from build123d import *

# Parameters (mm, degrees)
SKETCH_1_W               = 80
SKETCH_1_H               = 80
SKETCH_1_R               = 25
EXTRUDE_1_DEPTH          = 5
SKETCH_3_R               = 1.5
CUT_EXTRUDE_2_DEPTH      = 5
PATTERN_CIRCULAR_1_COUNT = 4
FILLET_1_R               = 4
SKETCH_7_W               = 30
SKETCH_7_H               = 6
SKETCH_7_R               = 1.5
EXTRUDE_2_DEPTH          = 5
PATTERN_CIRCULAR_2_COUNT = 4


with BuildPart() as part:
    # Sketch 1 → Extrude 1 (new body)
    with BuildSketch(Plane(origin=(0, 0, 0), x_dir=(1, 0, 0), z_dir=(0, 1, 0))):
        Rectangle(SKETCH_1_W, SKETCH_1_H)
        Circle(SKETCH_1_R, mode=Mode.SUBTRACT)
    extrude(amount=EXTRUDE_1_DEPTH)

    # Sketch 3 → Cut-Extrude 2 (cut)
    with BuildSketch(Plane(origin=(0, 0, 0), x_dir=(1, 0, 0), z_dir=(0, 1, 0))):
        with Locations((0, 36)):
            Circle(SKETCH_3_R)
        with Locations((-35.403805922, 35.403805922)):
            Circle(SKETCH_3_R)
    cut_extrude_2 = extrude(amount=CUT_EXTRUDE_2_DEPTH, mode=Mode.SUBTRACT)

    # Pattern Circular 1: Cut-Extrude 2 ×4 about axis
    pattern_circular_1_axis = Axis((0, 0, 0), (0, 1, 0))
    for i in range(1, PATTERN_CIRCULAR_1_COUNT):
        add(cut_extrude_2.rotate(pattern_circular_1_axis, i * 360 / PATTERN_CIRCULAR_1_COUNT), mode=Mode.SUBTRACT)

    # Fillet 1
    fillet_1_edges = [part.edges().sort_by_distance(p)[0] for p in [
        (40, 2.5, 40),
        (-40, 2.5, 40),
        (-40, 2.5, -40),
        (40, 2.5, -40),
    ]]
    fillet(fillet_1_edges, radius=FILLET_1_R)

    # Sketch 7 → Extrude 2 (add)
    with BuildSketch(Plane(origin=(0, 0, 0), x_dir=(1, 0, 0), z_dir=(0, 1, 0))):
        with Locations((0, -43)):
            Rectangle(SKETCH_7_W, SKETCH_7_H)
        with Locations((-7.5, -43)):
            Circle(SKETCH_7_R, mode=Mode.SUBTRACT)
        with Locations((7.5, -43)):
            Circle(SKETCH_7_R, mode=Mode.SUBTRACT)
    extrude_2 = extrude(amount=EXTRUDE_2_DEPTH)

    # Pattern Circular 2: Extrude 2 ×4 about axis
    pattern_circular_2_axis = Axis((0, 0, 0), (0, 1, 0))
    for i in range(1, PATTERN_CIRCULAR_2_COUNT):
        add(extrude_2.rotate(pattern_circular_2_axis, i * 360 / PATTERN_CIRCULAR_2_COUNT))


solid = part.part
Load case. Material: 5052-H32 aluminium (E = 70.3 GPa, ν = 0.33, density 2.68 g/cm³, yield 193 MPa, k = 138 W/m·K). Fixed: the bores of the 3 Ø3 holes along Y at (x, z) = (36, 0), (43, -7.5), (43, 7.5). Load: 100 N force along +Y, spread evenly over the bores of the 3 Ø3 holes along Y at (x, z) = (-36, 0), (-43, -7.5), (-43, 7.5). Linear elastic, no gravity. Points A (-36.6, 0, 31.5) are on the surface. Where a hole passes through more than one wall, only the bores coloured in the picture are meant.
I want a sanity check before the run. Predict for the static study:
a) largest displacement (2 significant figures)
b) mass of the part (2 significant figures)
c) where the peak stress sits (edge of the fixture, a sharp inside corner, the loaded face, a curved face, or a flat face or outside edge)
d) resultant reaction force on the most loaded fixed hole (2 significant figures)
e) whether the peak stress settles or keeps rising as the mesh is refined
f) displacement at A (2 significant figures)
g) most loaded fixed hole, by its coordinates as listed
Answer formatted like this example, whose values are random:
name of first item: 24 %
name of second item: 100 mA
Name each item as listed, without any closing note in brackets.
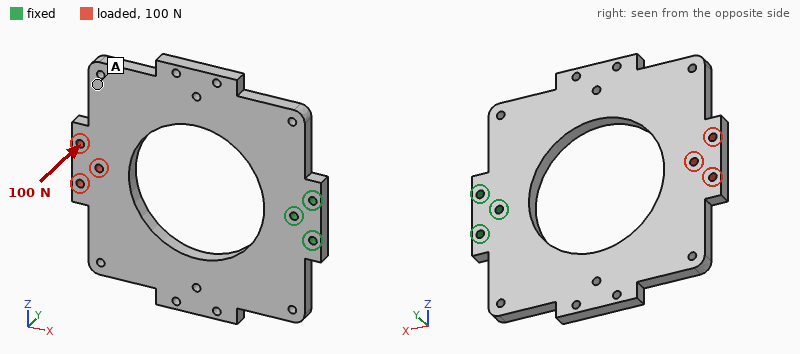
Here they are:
largest displacement: 0.77 mm
mass of the part: 67 g
where the peak stress sits: edge of the fixture
resultant reaction force on the most loaded fixed hole: 510 N
whether the peak stress settles or keeps rising as the mesh is refined: keeps rising
displacement at A: 0.64 mm
most loaded fixed hole, by its coordinates as listed: (36, 0)
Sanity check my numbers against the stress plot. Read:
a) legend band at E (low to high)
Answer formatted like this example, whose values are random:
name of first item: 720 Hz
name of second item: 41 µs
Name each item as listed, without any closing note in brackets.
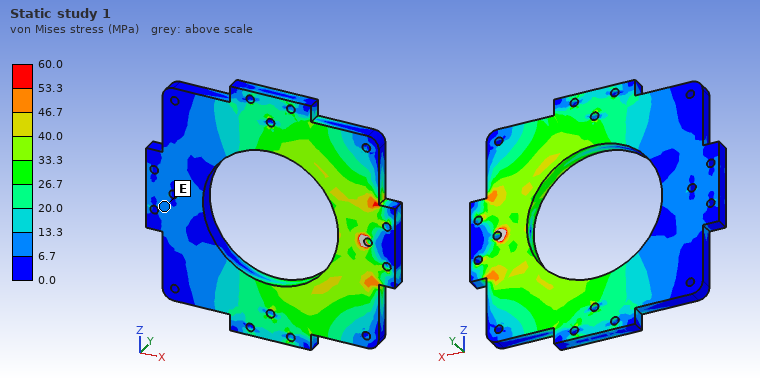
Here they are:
legend band at E: 6.7 to 13.3 MPa
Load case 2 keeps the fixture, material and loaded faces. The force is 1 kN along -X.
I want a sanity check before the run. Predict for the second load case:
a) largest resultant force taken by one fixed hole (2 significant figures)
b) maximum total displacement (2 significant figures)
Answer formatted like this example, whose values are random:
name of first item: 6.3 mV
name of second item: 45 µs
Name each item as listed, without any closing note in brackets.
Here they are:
largest resultant force taken by one fixed hole: 670 N
maximum total displacement: 35 µm
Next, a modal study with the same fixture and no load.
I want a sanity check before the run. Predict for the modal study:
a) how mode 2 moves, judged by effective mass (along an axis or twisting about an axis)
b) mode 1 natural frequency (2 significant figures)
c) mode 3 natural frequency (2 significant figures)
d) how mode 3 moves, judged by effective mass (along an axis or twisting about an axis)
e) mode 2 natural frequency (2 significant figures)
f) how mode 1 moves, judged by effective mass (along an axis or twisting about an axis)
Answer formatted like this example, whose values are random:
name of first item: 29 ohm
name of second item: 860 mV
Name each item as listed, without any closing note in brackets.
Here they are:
how mode 2 moves, judged by effective mass: twisting about X
mode 1 natural frequency: 430 Hz
mode 3 natural frequency: 1700 Hz
how mode 3 moves, judged by effective mass: along Z
mode 2 natural frequency: 820 Hz
how mode 1 moves, judged by effective mass: along Y
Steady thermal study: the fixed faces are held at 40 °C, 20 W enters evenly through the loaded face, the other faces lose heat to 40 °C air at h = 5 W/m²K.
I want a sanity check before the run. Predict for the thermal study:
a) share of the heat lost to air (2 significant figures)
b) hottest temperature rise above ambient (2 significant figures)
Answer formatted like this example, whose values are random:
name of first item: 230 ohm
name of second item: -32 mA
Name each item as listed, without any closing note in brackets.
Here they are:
share of the heat lost to air: 11 %
hottest temperature rise above ambient: 72 K
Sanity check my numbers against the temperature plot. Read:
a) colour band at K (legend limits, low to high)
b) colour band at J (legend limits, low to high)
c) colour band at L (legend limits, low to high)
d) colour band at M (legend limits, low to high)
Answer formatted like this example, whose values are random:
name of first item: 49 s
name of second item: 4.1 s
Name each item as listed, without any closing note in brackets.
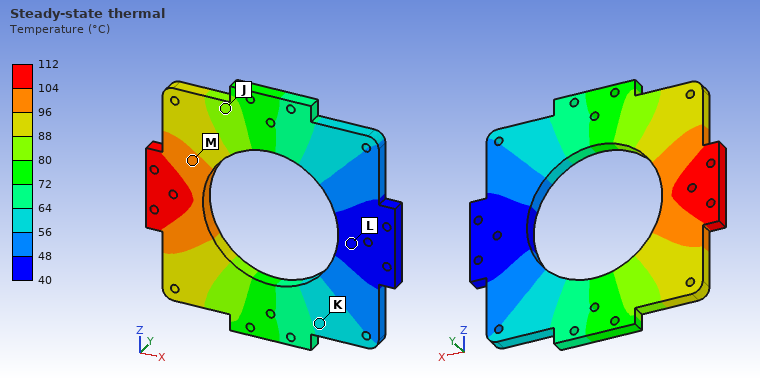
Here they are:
colour band at K: 56 to 64 °C
colour band at J: 80 to 88 °C
colour band at L: 40 to 48 °C
colour band at M: 96 to 104 °C
